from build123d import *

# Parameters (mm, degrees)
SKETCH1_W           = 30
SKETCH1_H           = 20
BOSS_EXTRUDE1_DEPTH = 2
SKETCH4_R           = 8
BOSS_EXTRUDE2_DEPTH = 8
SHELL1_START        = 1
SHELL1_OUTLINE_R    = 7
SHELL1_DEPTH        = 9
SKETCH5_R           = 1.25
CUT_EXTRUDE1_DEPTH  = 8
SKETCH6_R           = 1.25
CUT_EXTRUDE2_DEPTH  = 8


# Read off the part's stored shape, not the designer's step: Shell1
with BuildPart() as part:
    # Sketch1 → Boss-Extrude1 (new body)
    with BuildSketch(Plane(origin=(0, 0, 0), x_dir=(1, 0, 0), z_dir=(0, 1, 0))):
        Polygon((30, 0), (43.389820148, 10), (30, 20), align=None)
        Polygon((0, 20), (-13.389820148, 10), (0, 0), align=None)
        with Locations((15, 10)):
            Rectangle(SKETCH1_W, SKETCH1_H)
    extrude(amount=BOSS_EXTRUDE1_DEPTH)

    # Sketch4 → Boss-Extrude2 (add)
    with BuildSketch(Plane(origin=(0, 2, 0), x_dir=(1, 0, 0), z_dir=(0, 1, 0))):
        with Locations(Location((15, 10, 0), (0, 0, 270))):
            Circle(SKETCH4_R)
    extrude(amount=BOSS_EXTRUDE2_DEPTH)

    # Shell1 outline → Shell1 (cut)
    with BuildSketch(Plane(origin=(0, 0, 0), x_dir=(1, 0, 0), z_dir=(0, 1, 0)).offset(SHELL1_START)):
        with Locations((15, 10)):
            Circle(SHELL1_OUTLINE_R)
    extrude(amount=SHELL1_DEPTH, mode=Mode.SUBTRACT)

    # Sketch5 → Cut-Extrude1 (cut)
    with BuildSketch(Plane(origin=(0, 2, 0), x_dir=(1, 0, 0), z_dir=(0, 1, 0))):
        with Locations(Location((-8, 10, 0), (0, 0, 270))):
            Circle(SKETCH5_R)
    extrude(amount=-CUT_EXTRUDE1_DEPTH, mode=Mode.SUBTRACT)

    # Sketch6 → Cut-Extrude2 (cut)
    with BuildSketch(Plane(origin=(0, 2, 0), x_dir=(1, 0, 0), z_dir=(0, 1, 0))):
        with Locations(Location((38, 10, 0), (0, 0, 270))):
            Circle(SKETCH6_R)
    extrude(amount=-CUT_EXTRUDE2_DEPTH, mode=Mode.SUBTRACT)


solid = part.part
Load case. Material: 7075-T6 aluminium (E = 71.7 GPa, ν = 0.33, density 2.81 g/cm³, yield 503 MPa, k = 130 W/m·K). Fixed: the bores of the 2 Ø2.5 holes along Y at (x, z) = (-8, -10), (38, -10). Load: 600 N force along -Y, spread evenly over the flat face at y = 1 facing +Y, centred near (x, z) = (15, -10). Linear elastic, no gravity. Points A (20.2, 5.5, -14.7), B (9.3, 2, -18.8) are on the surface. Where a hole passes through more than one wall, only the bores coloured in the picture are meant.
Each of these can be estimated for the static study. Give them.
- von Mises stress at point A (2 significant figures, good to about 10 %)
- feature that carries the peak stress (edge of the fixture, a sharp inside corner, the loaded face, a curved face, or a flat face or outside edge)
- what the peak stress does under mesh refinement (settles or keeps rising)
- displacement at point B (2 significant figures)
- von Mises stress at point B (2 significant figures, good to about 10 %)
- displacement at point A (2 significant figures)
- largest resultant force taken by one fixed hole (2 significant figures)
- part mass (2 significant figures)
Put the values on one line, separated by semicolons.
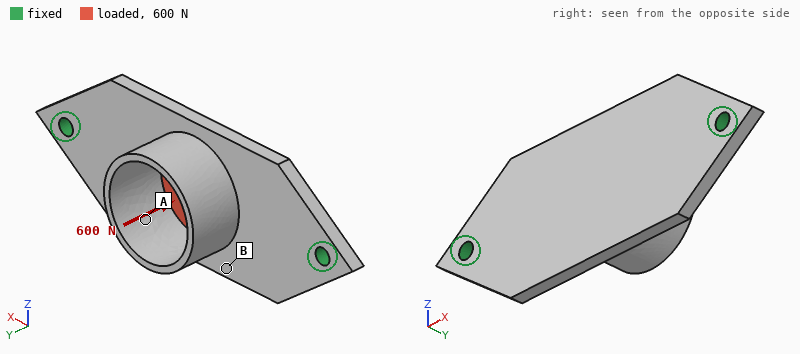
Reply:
54 MPa; edge of the fixture; keeps rising; 0.28 mm; 150 MPa; 0.28 mm; 330 N; 5.4 g
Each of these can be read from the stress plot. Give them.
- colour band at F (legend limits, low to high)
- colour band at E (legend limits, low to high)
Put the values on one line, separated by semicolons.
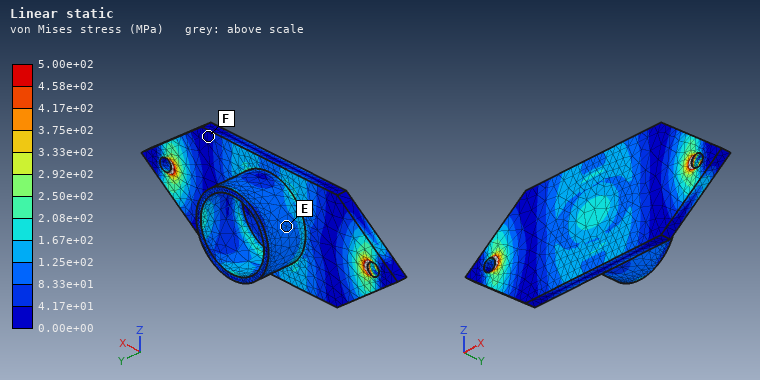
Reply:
0.00e+00 to 4.17e+01 MPa; 8.33e+01 to 1.25e+02 MPa
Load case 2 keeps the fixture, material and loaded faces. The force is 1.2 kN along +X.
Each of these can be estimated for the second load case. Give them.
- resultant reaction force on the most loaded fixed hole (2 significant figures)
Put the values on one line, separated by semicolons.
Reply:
600 N
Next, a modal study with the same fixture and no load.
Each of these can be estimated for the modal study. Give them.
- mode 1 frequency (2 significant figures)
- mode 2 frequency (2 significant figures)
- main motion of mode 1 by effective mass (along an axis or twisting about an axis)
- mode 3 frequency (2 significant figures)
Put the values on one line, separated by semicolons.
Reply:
4100 Hz; 4600 Hz; along Y; 10000 Hz
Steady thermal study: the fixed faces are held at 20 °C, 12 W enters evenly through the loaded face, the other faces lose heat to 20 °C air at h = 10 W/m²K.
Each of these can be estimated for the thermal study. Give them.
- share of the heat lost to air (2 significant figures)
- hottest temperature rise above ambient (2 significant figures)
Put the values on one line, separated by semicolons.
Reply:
4.5 %; 35 K
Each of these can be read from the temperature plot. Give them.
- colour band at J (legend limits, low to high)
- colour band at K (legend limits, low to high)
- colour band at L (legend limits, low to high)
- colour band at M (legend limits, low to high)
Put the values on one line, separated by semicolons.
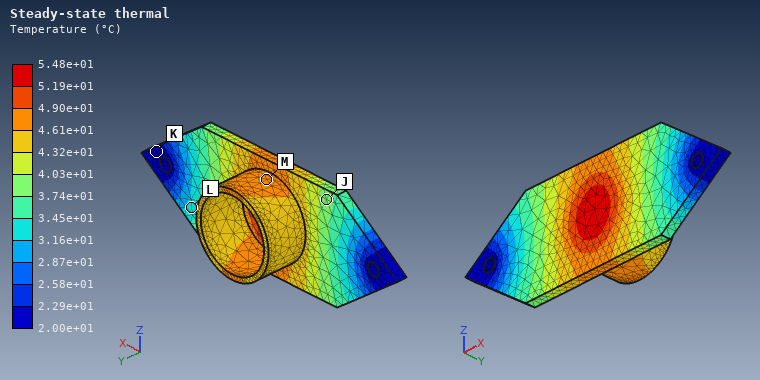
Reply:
3.74e+01 to 4.03e+01 °C; 2.00e+01 to 2.29e+01 °C; 3.16e+01 to 3.45e+01 °C; 4.61e+01 to 4.90e+01 °C
